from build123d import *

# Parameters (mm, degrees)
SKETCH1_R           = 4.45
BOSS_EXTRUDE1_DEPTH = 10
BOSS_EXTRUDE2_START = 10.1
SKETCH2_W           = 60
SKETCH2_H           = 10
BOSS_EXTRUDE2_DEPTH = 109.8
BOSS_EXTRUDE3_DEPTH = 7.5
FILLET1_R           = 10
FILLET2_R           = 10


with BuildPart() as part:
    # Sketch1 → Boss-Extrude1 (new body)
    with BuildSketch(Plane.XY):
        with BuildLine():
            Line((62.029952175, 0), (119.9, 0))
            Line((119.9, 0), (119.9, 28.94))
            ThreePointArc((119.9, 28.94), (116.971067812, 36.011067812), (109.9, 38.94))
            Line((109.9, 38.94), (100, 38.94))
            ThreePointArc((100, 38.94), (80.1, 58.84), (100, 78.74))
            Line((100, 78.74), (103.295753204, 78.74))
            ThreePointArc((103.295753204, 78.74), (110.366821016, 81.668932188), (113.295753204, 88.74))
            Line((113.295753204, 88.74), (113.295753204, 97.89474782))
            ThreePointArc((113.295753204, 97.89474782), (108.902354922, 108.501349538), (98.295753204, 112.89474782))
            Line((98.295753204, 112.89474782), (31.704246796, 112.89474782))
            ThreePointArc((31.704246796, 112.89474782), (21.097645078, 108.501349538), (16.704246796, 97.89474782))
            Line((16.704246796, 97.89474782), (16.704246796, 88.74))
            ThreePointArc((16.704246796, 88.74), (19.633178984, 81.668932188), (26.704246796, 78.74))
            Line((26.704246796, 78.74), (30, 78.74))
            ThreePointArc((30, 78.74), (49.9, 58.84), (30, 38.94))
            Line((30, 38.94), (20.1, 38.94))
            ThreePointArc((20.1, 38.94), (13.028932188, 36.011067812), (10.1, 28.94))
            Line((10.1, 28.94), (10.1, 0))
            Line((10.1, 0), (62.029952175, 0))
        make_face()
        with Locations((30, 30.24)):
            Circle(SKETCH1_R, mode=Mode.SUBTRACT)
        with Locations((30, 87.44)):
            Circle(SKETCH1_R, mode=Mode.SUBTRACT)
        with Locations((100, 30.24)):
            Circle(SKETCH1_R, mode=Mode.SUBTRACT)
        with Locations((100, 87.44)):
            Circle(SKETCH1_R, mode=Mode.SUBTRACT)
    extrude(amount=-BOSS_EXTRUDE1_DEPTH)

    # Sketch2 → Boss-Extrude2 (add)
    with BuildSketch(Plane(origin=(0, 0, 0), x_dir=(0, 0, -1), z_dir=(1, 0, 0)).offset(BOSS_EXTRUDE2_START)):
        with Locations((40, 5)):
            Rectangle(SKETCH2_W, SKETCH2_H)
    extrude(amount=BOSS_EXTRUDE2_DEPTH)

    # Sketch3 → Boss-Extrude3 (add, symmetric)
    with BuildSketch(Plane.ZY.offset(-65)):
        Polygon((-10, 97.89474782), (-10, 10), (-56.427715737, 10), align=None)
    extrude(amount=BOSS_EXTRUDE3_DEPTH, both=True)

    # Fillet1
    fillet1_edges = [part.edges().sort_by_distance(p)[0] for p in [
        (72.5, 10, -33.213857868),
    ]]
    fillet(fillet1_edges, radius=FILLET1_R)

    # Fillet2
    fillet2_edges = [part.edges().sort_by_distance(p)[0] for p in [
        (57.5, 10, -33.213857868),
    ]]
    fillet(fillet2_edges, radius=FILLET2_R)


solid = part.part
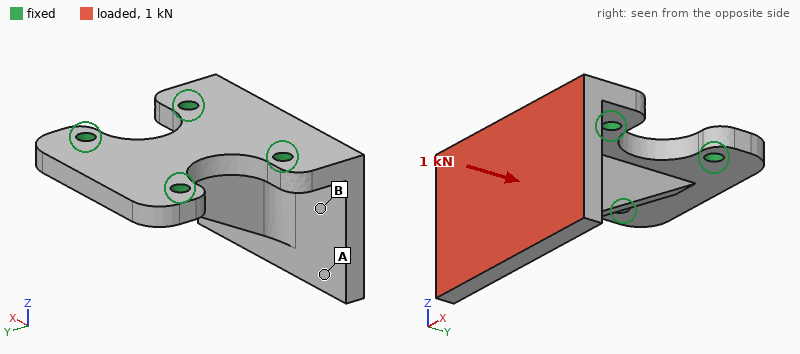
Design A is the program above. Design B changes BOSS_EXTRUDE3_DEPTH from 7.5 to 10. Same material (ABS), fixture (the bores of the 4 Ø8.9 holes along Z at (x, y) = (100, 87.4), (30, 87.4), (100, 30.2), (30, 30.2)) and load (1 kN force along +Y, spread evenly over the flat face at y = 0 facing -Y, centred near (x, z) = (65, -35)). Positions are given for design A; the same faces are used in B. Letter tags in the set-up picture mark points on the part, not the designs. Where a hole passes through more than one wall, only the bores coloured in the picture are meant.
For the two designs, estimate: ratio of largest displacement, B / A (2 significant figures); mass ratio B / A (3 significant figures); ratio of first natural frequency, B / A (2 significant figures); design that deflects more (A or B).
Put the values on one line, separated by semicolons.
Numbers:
0.89; 1.06; 1.0; A
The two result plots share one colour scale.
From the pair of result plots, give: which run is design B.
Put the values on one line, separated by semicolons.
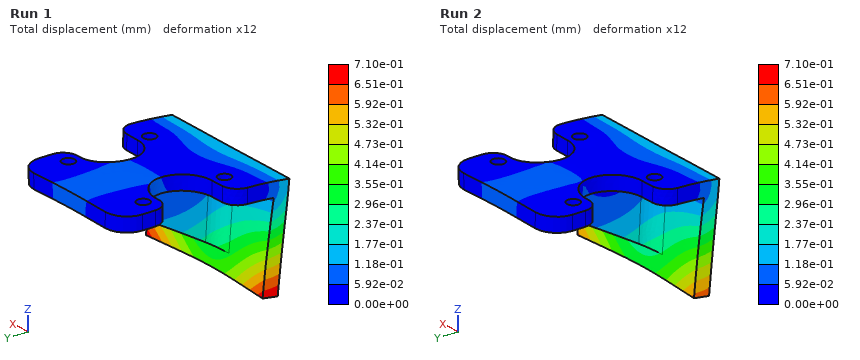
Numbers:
Run 2
